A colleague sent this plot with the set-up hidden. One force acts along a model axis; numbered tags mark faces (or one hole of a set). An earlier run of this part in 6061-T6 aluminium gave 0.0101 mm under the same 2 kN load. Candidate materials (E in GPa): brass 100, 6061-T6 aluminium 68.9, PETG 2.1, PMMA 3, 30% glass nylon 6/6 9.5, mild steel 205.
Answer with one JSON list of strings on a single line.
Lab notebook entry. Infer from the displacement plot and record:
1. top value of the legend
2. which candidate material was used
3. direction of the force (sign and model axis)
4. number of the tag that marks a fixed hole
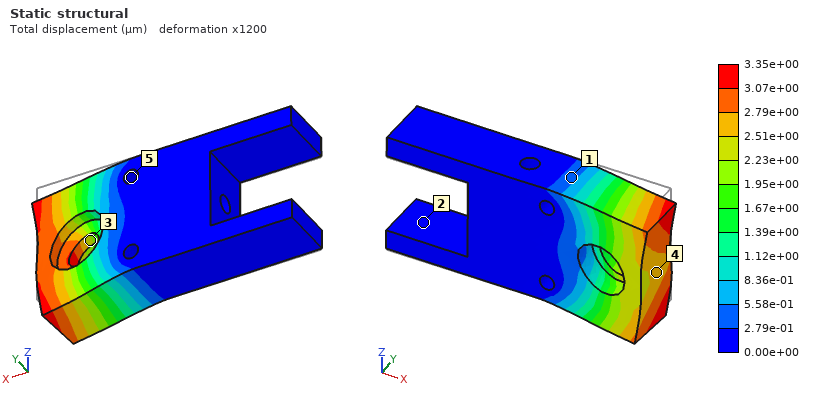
["3.35e+00 µm", "mild steel", "-Z", "5"]
